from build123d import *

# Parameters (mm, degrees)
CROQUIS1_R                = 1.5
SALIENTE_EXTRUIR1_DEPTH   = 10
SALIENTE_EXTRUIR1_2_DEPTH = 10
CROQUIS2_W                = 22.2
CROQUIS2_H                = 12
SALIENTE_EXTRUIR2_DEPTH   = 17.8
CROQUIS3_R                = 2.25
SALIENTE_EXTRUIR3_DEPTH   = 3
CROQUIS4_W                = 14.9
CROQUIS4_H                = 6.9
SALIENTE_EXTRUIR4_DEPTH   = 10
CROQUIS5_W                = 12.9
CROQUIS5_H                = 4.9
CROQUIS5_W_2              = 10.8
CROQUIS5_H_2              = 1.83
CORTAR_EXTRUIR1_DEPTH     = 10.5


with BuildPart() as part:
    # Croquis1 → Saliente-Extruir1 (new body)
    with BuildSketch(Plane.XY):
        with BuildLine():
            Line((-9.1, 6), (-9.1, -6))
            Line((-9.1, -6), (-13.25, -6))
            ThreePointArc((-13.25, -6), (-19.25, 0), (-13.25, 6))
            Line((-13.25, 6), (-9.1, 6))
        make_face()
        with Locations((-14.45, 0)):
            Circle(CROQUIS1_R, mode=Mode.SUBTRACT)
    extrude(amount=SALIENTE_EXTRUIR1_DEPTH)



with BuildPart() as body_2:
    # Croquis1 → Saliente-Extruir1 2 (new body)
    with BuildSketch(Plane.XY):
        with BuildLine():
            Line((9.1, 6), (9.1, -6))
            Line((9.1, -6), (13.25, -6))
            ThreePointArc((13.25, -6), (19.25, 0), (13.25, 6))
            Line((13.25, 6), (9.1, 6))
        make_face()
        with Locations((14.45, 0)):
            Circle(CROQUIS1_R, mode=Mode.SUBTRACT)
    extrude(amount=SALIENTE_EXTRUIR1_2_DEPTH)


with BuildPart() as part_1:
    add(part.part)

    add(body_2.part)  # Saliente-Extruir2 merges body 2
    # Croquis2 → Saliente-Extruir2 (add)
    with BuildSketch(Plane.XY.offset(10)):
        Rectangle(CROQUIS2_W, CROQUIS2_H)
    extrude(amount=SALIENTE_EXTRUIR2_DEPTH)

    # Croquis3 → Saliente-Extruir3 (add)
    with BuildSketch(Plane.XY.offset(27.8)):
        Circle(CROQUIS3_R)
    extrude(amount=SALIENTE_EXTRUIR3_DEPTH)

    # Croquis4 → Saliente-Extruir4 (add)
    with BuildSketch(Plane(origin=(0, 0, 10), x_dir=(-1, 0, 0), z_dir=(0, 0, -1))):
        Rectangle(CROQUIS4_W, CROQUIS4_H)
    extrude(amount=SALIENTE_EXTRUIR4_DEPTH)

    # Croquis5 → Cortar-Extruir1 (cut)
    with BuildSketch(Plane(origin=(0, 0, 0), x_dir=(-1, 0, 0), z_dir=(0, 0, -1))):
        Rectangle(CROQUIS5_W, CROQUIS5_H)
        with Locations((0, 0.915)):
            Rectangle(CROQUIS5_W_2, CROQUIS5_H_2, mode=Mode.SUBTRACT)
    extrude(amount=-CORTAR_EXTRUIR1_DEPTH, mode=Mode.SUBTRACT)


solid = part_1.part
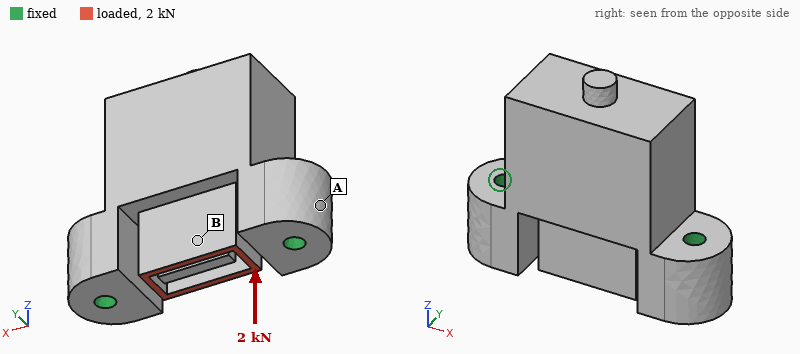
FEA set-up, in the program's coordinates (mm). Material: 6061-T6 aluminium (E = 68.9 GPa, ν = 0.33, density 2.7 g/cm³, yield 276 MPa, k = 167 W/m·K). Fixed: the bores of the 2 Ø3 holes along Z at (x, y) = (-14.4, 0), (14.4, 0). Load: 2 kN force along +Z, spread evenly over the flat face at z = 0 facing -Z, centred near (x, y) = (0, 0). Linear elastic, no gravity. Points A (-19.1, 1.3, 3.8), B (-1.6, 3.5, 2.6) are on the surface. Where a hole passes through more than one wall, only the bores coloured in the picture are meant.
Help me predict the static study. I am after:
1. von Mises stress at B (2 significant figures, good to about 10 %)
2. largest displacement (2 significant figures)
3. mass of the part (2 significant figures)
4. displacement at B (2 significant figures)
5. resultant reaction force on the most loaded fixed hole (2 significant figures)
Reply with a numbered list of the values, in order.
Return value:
1. 48 MPa
2. 14 µm
3. 20 g
4. 12 µm
5. 1.1 kN
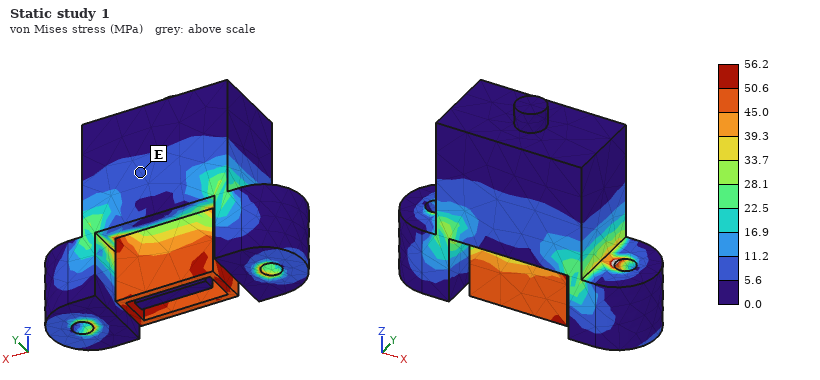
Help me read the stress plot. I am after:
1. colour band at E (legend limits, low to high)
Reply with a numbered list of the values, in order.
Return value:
1. 5.6 to 11.2 MPa
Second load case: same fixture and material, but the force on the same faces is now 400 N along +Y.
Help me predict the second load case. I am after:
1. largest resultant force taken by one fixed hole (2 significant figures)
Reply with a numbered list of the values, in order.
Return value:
1. 200 N
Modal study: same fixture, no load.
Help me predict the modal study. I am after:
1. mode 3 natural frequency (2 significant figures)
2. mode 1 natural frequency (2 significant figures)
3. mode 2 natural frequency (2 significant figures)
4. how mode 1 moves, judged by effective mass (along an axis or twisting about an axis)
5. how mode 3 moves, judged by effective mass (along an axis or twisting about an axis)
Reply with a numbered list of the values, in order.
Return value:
1. 20 kHz
2. 7600 Hz
3. 12 kHz
4. along Y
5. along X
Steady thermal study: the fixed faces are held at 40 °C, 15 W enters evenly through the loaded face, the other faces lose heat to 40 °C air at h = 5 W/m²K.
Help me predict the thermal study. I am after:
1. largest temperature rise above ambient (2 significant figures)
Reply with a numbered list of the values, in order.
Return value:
1. 33 K
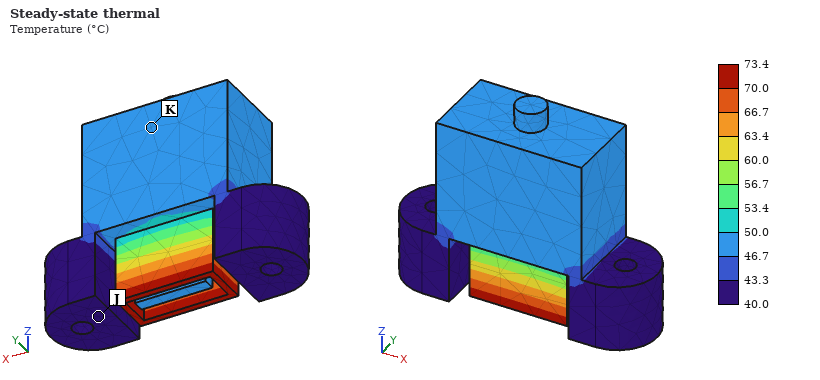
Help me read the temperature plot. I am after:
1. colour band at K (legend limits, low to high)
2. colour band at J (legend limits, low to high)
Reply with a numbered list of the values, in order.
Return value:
1. 46.7 to 50.0 °C
2. 40.0 to 43.3 °C
